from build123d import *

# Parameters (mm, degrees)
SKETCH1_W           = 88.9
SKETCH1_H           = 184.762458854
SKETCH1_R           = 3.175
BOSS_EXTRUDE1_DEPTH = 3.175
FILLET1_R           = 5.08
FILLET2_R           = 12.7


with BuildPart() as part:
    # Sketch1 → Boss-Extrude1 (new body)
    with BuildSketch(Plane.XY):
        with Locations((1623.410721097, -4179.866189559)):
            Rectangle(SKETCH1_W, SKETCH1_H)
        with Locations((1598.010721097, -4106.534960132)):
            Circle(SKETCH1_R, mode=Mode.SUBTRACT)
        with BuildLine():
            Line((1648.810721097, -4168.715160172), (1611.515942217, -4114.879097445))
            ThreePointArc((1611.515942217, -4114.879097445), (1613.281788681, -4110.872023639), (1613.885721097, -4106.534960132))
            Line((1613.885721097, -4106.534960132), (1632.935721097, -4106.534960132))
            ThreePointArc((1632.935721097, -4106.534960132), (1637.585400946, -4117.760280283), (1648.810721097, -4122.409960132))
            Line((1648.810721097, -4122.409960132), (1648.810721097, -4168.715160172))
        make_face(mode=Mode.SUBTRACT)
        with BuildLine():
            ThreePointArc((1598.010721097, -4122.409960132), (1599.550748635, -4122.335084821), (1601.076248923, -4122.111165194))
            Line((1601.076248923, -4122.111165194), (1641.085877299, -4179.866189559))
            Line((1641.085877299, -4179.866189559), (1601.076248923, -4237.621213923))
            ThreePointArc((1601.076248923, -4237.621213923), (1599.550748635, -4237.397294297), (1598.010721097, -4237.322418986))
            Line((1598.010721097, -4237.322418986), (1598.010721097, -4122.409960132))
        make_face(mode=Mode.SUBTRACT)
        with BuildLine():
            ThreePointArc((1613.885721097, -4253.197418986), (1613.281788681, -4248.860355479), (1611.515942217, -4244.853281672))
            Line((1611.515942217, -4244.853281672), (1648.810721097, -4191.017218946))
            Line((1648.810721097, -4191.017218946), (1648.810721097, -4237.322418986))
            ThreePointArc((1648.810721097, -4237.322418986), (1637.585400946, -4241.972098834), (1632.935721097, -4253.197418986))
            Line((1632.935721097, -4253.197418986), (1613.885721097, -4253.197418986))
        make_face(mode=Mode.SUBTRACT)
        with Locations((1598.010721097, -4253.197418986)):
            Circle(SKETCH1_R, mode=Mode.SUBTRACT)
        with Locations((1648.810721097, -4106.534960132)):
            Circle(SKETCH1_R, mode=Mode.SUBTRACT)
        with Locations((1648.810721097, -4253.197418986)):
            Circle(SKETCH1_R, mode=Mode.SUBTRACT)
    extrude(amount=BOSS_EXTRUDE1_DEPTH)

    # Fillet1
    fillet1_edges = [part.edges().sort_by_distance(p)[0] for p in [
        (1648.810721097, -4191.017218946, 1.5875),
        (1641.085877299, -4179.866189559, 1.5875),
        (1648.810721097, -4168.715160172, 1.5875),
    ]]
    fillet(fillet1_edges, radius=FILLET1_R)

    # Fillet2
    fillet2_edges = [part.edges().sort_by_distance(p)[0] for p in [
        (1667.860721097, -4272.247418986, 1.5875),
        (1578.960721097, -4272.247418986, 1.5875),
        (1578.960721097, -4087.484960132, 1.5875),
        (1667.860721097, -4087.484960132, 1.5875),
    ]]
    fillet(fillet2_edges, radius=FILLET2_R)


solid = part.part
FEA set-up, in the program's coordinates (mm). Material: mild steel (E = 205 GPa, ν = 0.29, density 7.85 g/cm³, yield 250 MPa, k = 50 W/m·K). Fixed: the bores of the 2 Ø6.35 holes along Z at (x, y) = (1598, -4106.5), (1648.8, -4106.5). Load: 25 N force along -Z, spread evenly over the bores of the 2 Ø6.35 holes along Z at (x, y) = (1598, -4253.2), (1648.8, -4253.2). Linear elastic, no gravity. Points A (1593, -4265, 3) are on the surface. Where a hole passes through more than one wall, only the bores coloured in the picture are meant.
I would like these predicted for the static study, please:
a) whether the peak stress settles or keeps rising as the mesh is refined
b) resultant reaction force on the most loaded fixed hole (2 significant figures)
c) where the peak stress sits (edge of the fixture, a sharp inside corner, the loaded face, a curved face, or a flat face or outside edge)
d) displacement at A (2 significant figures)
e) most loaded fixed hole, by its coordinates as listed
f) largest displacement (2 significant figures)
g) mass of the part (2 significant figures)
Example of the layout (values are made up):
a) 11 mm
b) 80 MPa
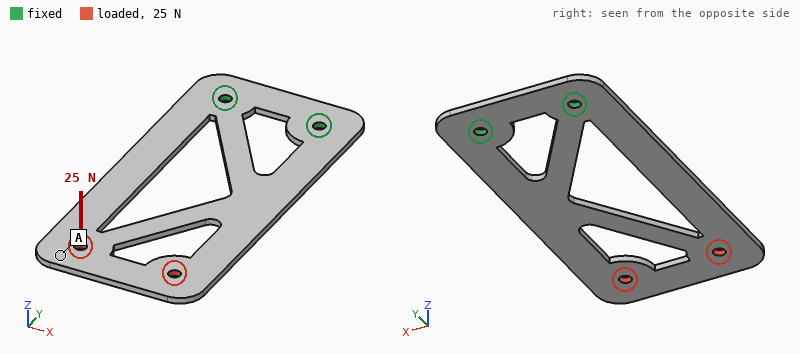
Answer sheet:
a) keeps rising
b) 15 N
c) edge of the fixture
d) 1.0 mm
e) (1598, -4106.5)
f) 1.1 mm
g) 280 g
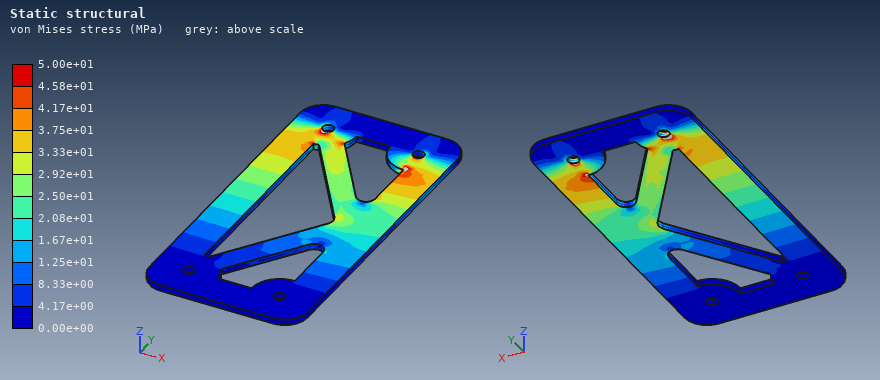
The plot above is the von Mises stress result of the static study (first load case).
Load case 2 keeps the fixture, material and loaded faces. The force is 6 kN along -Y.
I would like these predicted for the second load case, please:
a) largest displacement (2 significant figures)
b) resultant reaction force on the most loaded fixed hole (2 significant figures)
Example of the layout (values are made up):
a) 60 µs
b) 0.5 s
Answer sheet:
a) 52 µm
b) 3.2 kN
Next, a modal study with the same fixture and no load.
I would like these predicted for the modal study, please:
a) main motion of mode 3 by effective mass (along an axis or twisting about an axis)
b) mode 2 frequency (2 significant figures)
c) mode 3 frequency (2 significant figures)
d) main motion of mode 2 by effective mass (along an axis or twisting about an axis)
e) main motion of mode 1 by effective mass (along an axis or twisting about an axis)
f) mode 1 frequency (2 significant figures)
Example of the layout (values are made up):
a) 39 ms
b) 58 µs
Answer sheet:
a) along Z
b) 310 Hz
c) 560 Hz
d) twisting about Y
e) along Z
f) 84 Hz
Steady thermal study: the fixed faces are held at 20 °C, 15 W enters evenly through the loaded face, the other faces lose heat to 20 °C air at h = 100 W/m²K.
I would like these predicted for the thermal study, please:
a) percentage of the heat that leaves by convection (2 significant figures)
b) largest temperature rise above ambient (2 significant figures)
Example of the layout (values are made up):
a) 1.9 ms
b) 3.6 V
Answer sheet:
a) 100 %
b) 30 K
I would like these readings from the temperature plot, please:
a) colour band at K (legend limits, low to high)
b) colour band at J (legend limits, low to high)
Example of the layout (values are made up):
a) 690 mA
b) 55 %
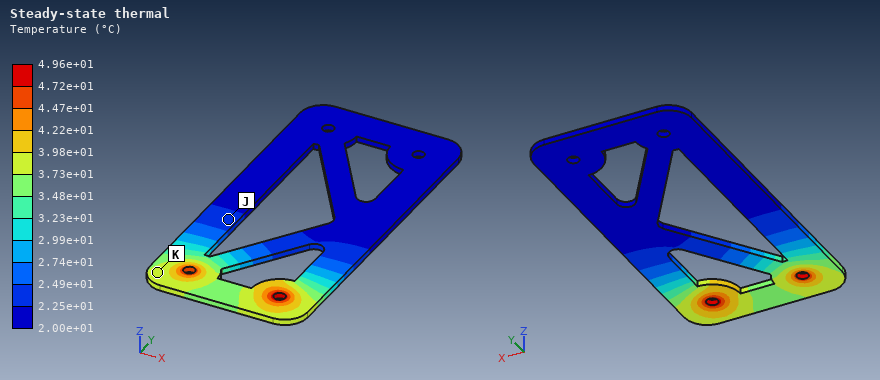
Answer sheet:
a) 3.73e+01 to 3.98e+01 °C
b) 2.25e+01 to 2.49e+01 °C
